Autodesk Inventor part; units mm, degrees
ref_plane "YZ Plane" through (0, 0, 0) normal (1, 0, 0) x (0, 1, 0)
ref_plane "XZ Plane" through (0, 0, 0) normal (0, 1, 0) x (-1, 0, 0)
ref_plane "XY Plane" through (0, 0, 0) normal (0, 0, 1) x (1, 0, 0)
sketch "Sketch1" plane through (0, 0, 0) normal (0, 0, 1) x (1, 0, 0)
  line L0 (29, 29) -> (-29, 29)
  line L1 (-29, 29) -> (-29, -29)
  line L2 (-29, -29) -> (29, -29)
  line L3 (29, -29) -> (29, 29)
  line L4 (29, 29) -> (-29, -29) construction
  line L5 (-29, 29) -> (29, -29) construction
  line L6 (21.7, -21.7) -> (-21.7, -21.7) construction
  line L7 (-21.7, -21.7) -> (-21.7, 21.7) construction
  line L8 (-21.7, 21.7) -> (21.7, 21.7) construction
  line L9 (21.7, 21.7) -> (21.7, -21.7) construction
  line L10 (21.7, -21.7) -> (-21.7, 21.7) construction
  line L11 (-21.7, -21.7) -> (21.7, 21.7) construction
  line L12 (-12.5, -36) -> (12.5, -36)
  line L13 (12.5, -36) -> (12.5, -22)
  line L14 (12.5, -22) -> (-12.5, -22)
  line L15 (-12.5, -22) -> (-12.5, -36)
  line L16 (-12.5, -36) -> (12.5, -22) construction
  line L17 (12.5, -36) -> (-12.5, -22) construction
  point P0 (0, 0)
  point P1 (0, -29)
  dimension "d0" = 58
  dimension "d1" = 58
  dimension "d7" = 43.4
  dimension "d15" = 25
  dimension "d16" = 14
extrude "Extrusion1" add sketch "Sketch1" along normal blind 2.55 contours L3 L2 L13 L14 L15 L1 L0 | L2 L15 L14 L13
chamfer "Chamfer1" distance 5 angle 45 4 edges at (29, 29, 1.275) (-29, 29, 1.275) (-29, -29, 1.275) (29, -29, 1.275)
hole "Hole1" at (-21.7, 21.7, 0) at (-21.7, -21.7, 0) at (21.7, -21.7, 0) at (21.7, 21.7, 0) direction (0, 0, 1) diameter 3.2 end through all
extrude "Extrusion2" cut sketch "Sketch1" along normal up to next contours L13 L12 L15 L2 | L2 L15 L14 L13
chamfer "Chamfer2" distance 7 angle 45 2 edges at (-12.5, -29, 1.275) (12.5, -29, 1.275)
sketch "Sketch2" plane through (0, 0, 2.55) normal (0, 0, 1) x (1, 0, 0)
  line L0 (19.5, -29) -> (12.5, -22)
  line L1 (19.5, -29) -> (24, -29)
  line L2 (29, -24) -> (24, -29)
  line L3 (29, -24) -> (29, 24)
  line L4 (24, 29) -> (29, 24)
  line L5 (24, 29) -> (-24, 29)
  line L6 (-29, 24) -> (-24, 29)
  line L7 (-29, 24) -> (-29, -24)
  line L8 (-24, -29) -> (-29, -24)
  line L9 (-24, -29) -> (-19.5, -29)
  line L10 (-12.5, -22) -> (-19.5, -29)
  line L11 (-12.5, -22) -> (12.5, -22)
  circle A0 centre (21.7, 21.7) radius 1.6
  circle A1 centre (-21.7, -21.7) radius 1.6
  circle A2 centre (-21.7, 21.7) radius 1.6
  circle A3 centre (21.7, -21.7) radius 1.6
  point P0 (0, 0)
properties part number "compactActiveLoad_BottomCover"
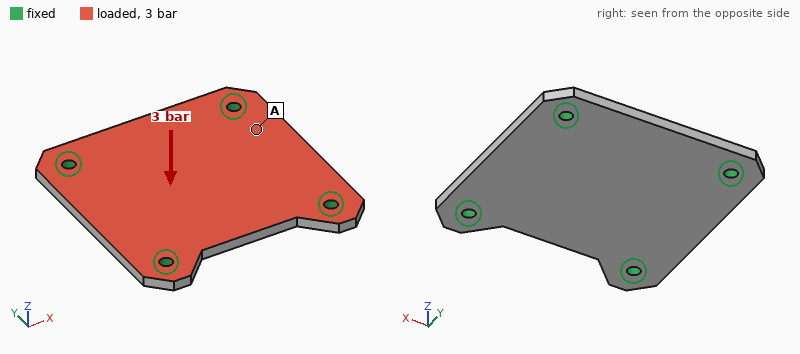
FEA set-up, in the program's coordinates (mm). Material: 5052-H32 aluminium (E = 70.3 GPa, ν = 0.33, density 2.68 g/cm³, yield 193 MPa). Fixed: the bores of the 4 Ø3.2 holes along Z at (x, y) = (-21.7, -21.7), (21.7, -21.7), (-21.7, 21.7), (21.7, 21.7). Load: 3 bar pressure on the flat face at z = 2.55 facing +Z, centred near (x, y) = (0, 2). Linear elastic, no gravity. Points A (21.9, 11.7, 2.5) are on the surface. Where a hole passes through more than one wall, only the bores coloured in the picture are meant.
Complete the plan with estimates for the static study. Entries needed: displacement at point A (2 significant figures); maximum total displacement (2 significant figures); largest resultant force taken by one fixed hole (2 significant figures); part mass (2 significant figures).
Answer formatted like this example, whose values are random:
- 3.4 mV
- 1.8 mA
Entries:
- 20 µm
- 68 µm
- 250 N
- 21 g
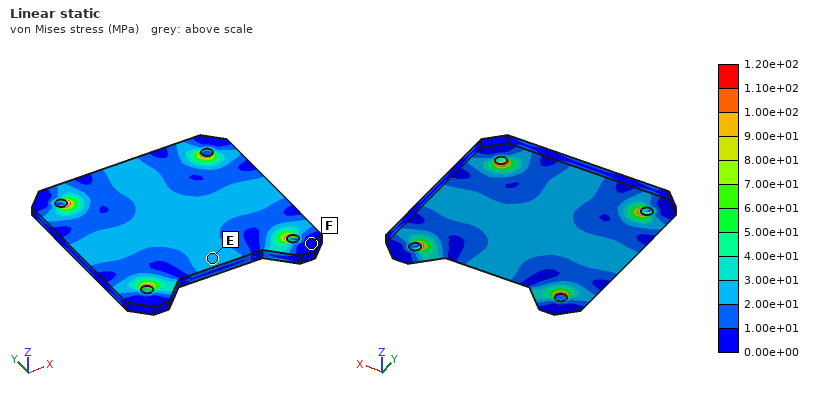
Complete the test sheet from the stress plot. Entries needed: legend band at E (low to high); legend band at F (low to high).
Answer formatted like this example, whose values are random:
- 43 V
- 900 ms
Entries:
- 2.00e+01 to 3.00e+01 MPa
- 0.00e+00 to 1.00e+01 MPa
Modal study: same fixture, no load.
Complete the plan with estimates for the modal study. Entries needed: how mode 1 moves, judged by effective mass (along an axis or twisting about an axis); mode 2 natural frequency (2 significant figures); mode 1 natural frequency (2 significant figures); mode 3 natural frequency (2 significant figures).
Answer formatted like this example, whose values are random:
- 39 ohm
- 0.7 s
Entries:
- along Z
- 7700 Hz
- 4900 Hz
- 7800 Hz
